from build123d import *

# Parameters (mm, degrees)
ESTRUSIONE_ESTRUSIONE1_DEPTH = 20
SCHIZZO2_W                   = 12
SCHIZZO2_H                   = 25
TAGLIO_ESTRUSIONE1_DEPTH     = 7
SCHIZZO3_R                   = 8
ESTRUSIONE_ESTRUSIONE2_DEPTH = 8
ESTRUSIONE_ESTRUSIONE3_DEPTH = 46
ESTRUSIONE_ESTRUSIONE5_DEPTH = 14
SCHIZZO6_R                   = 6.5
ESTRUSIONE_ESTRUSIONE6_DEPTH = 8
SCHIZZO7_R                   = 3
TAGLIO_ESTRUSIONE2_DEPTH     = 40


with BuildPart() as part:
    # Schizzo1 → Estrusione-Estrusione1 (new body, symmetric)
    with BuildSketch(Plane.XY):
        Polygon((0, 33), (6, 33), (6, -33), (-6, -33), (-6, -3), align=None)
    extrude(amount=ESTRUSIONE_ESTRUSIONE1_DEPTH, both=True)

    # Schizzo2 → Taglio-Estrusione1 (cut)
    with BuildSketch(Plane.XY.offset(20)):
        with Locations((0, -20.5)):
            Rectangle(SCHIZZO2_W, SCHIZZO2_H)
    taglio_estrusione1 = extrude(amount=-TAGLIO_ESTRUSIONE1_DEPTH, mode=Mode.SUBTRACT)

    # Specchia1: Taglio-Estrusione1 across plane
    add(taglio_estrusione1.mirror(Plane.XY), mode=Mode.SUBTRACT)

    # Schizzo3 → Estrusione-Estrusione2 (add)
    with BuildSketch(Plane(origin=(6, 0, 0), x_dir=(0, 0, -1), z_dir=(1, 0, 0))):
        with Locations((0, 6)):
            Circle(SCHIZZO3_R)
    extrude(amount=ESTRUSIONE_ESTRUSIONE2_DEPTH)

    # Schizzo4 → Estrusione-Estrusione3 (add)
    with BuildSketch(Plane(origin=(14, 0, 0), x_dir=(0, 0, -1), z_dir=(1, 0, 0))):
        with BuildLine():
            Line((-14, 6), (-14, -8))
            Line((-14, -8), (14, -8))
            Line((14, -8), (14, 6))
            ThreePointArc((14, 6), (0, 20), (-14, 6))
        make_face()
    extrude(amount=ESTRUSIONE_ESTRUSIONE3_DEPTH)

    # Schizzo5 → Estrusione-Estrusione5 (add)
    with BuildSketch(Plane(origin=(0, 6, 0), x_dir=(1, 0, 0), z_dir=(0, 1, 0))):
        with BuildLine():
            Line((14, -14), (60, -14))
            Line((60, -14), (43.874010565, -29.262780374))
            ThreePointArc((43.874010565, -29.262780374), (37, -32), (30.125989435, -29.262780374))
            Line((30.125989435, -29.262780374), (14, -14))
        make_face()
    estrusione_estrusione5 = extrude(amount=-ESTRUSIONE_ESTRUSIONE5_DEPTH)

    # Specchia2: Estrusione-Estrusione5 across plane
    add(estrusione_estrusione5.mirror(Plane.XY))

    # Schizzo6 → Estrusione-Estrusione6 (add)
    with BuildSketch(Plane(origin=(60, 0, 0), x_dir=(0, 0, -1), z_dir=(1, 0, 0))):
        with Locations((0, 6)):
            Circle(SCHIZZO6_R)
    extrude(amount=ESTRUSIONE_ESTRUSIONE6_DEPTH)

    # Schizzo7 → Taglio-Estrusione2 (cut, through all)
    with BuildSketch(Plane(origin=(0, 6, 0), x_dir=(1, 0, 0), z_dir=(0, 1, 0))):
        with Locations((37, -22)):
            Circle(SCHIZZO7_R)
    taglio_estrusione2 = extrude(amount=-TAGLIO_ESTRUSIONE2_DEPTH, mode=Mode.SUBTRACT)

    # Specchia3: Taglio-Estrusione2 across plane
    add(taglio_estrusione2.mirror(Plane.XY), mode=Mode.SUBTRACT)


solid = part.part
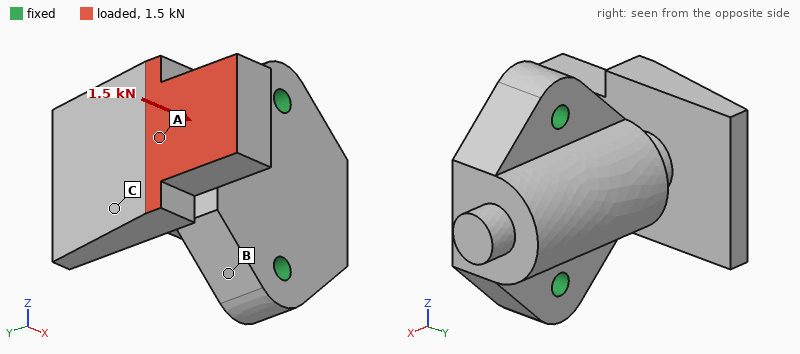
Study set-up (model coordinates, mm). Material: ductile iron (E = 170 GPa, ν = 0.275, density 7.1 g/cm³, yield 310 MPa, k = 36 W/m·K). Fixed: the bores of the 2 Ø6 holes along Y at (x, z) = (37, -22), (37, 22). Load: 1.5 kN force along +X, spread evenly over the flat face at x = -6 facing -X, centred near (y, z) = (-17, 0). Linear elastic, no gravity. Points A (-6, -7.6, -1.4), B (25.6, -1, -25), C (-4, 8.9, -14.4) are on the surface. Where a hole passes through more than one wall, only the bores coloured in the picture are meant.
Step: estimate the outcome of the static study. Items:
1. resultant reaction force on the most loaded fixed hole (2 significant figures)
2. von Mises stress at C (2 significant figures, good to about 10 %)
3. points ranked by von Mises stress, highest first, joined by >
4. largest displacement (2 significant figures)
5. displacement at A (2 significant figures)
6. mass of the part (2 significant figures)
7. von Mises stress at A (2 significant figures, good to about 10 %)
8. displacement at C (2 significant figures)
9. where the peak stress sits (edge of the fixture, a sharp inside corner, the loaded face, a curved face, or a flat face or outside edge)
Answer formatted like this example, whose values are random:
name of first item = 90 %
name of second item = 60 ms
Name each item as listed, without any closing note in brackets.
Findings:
resultant reaction force on the most loaded fixed hole = 820 N
von Mises stress at C = 11 MPa
points ranked by von Mises stress, highest first, joined by > = A > C > B
largest displacement = 63 µm
displacement at A = 30 µm
mass of the part = 500 g
von Mises stress at A = 20 MPa
displacement at C = 20 µm
where the peak stress sits = a curved face
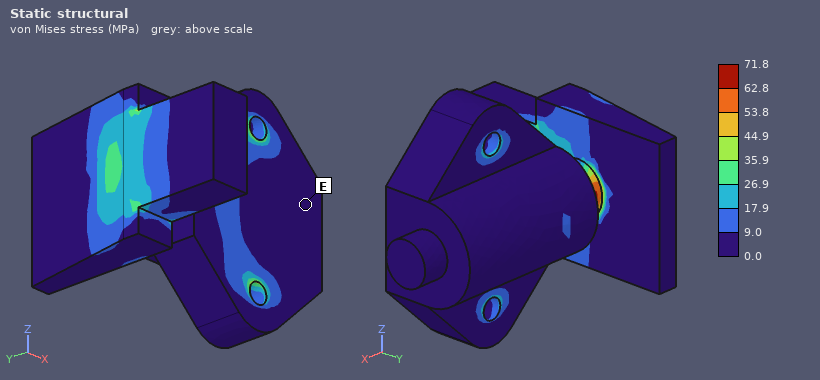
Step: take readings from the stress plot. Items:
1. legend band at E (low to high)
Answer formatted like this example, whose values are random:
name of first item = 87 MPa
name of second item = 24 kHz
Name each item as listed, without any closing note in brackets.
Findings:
legend band at E = 0.0 to 9.0 MPa
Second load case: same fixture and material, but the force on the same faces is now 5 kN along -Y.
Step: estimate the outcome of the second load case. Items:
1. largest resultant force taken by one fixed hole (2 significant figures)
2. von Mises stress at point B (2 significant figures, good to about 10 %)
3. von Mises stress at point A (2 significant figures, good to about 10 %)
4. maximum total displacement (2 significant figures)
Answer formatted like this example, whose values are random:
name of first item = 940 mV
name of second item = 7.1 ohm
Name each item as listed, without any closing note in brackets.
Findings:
largest resultant force taken by one fixed hole = 2.9 kN
von Mises stress at point B = 54 MPa
von Mises stress at point A = 46 MPa
maximum total displacement = 0.18 mm
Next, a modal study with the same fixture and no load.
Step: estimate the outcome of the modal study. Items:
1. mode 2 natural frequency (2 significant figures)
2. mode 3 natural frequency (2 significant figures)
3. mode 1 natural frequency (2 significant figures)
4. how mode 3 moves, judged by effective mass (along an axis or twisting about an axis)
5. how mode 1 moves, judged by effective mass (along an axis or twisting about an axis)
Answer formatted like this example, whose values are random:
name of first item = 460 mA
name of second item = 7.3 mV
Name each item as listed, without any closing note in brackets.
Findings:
mode 2 natural frequency = 3100 Hz
mode 3 natural frequency = 4800 Hz
mode 1 natural frequency = 2600 Hz
how mode 3 moves, judged by effective mass = along Z
how mode 1 moves, judged by effective mass = along Y
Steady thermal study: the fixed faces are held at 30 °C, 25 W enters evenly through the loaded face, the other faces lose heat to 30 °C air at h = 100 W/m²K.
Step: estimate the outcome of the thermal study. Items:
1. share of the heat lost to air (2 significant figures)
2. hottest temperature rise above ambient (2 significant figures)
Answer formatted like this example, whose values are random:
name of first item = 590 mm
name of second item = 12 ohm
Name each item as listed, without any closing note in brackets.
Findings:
share of the heat lost to air = 75 %
hottest temperature rise above ambient = 52 K
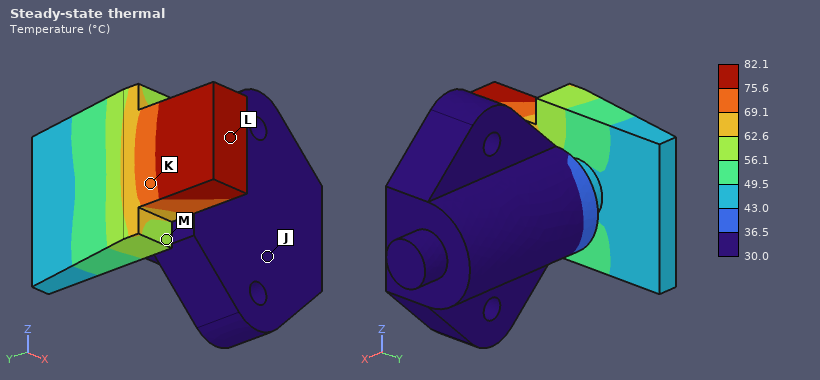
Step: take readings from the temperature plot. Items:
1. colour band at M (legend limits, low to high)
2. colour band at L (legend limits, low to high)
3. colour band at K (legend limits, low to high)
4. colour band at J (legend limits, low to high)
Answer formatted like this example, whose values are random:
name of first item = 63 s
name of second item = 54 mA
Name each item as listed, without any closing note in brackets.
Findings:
colour band at M = 56.1 to 62.6 °C
colour band at L = 75.6 to 82.1 °C
colour band at K = 69.1 to 75.6 °C
colour band at J = 30.0 to 36.5 °C
